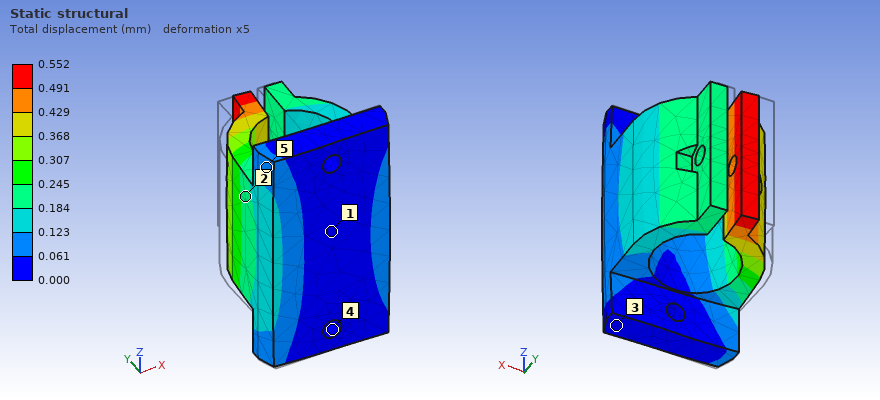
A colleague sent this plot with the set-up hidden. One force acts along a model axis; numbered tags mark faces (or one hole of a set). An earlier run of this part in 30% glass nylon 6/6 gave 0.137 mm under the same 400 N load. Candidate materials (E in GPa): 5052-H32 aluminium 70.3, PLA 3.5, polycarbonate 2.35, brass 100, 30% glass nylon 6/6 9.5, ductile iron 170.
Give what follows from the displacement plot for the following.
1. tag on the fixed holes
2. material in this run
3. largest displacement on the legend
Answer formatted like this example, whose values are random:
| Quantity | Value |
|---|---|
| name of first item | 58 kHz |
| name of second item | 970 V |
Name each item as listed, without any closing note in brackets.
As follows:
| Quantity | Value |
|---|---|
| tag on the fixed holes | 4 |
| material in this run | polycarbonate |
| largest displacement on the legend | 0.552 mm |
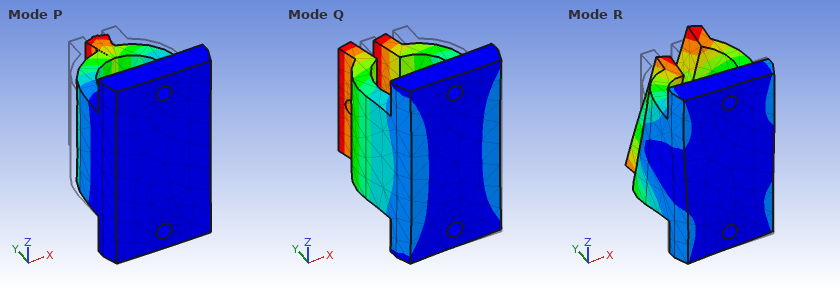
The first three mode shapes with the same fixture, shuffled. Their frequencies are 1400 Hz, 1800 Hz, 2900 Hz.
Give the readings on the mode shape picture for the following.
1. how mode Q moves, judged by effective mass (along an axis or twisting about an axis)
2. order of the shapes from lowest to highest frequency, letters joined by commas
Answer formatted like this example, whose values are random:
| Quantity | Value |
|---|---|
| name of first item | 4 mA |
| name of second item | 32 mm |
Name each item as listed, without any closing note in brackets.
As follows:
| Quantity | Value |
|---|---|
| how mode Q moves, judged by effective mass | along X |
| order of the shapes from lowest to highest frequency, letters joined by commas | Q, P, R |
